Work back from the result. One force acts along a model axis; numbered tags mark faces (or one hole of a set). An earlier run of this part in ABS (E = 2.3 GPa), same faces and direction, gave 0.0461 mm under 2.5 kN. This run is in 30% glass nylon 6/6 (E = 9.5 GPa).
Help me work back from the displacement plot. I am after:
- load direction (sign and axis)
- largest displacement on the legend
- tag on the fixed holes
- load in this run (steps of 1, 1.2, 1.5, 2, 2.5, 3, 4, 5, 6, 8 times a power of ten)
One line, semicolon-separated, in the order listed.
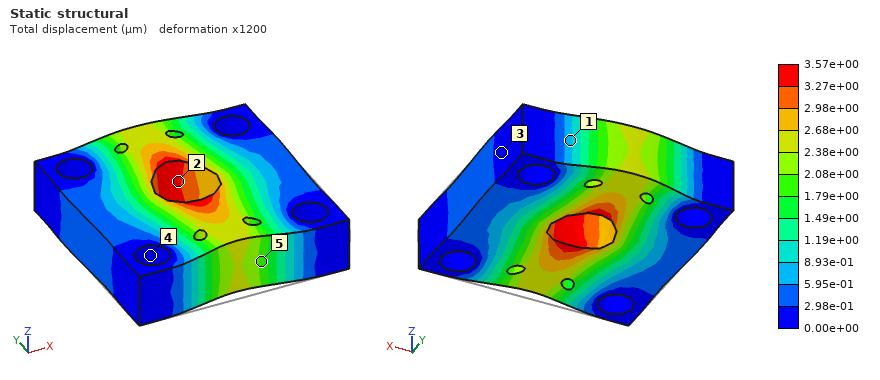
+Y; 3.57e+00 µm; 4; 800 N
